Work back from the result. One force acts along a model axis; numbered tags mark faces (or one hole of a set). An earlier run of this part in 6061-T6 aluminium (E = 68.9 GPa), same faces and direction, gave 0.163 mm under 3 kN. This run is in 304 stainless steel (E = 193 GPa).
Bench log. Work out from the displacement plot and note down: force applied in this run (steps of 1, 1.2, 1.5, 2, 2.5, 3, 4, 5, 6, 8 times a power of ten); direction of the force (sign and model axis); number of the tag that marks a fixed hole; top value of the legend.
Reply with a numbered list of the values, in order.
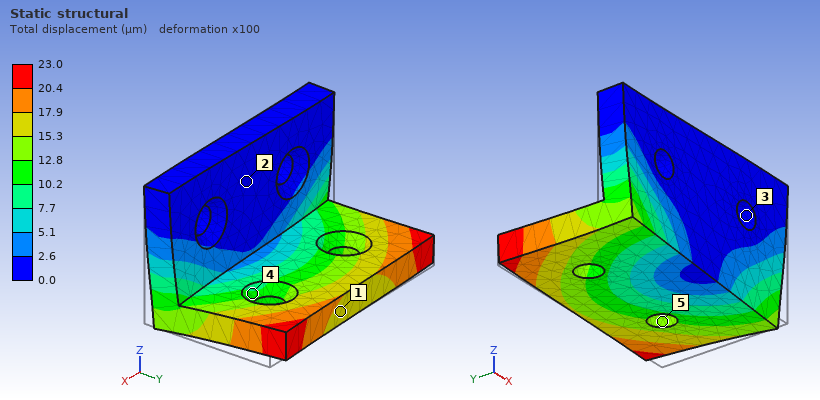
1. 1.2 kN
2. -X
3. 3
4. 23.0 µm
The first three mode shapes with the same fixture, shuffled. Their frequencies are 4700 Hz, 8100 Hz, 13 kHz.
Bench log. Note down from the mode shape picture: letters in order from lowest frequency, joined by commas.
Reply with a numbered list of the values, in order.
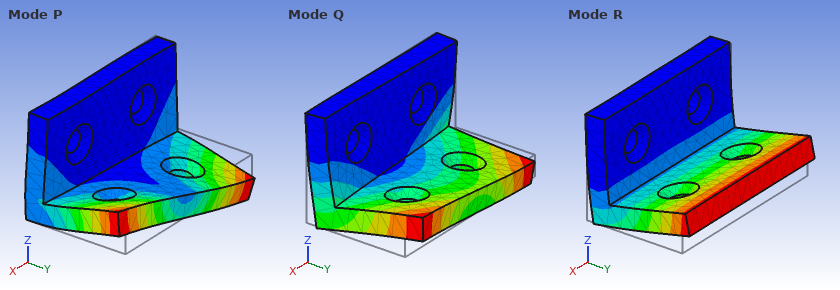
1. R, Q, P
